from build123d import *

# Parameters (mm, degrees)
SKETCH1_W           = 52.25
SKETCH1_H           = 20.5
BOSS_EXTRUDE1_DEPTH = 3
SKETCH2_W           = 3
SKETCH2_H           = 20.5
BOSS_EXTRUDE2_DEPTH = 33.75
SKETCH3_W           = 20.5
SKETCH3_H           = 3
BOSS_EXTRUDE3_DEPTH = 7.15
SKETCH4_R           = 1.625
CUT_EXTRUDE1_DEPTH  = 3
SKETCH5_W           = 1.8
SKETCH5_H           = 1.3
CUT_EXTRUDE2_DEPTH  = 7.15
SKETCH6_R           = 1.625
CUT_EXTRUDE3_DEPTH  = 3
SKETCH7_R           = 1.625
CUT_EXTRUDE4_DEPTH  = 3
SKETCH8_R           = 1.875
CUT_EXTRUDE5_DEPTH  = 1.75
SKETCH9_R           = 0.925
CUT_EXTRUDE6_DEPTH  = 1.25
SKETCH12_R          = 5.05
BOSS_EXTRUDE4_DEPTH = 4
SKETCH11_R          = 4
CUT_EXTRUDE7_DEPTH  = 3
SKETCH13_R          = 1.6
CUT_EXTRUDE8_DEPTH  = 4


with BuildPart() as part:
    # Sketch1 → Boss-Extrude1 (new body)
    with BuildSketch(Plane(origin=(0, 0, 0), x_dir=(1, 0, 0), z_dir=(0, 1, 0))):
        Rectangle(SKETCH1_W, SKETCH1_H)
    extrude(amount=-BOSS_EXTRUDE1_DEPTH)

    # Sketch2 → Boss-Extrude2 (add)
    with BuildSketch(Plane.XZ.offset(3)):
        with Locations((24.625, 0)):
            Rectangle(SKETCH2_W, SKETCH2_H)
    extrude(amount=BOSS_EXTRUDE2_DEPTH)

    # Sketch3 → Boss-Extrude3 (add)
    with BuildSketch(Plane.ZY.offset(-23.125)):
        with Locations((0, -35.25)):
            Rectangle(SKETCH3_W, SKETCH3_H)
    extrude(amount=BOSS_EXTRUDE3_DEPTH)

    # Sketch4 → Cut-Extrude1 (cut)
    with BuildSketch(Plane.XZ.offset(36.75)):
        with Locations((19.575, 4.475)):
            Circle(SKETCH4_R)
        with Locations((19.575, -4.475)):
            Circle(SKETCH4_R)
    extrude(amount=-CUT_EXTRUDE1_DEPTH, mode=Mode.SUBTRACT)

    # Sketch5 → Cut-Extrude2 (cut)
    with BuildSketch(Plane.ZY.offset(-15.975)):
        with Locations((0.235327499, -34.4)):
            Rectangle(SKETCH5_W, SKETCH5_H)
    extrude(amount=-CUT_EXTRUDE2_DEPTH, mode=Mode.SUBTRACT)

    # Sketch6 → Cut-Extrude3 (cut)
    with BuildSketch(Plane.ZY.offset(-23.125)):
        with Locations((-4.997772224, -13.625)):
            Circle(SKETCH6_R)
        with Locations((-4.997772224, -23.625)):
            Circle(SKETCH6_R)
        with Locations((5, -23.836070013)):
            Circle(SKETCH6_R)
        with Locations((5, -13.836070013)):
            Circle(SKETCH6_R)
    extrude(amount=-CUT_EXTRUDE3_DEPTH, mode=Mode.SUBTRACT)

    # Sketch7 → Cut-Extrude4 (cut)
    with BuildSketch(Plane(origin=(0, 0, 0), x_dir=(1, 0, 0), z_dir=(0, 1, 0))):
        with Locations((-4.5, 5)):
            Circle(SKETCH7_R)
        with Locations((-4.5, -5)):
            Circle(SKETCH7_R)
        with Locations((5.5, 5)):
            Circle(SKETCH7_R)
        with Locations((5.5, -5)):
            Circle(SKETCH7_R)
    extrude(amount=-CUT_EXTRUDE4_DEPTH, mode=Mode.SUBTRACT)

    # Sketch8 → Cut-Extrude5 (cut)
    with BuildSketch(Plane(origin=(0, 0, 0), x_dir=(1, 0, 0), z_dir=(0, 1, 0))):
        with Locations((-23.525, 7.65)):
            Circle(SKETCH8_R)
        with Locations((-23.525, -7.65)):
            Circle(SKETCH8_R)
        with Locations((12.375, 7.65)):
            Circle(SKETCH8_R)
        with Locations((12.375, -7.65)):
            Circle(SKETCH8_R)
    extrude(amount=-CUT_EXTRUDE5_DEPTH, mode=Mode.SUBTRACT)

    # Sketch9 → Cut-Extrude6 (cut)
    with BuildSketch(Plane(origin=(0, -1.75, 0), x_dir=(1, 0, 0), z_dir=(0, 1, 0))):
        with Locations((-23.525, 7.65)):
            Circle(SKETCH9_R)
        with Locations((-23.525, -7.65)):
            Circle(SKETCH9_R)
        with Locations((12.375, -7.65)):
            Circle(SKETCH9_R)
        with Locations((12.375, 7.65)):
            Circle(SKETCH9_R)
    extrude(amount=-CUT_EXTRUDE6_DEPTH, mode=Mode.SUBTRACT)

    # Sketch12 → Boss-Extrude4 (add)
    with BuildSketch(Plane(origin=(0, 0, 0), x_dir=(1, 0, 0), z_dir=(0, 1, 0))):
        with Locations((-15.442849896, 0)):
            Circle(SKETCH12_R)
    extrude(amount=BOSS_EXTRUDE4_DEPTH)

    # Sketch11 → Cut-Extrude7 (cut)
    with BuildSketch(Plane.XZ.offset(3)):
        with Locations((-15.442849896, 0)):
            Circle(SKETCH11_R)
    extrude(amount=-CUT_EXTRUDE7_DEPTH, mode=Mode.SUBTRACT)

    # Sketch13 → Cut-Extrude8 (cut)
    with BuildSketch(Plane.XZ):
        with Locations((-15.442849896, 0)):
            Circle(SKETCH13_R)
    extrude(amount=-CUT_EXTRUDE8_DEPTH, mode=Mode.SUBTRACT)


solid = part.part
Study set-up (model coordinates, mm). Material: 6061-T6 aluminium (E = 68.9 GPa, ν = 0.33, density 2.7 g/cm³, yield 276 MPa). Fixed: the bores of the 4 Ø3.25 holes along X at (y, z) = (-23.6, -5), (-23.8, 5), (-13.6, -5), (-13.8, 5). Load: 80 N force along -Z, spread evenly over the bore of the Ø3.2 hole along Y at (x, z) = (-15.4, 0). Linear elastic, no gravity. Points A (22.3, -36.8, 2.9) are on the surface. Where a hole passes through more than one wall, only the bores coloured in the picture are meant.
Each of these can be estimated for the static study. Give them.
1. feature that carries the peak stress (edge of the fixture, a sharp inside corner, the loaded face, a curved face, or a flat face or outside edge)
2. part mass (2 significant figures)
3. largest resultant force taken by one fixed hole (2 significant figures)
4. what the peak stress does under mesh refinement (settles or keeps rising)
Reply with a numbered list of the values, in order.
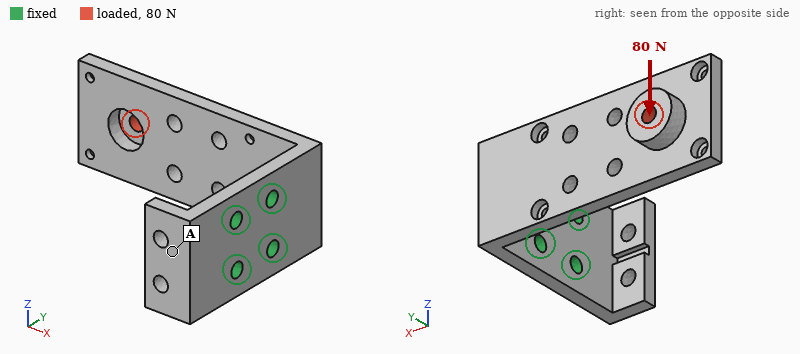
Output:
1. edge of the fixture
2. 15 g
3. 270 N
4. keeps rising
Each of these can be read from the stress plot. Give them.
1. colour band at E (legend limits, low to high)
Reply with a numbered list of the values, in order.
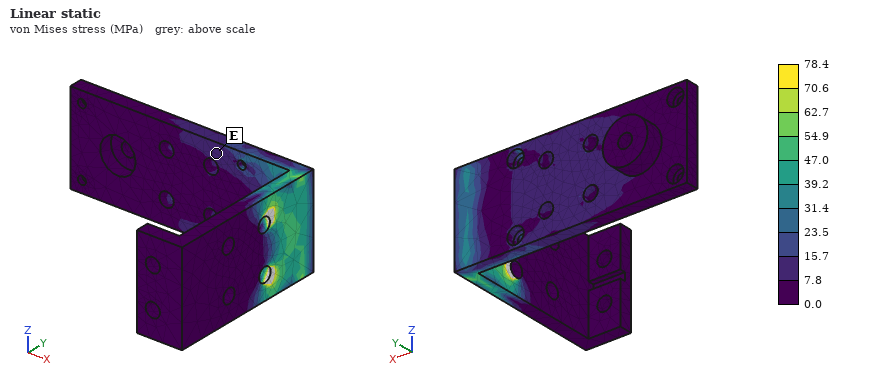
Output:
1. 7.8 to 15.7 MPa
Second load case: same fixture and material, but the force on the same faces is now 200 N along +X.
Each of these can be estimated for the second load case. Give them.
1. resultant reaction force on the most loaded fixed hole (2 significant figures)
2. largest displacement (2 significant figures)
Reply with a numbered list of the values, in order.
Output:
1. 130 N
2. 0.62 mm
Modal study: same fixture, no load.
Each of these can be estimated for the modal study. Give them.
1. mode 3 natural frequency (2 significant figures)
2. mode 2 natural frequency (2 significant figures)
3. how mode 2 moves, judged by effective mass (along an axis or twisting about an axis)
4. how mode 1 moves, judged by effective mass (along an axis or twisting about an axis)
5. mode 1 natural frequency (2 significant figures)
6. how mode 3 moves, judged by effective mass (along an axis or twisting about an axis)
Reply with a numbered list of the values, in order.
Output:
1. 4100 Hz
2. 1600 Hz
3. along Z
4. along Y
5. 680 Hz
6. along X
